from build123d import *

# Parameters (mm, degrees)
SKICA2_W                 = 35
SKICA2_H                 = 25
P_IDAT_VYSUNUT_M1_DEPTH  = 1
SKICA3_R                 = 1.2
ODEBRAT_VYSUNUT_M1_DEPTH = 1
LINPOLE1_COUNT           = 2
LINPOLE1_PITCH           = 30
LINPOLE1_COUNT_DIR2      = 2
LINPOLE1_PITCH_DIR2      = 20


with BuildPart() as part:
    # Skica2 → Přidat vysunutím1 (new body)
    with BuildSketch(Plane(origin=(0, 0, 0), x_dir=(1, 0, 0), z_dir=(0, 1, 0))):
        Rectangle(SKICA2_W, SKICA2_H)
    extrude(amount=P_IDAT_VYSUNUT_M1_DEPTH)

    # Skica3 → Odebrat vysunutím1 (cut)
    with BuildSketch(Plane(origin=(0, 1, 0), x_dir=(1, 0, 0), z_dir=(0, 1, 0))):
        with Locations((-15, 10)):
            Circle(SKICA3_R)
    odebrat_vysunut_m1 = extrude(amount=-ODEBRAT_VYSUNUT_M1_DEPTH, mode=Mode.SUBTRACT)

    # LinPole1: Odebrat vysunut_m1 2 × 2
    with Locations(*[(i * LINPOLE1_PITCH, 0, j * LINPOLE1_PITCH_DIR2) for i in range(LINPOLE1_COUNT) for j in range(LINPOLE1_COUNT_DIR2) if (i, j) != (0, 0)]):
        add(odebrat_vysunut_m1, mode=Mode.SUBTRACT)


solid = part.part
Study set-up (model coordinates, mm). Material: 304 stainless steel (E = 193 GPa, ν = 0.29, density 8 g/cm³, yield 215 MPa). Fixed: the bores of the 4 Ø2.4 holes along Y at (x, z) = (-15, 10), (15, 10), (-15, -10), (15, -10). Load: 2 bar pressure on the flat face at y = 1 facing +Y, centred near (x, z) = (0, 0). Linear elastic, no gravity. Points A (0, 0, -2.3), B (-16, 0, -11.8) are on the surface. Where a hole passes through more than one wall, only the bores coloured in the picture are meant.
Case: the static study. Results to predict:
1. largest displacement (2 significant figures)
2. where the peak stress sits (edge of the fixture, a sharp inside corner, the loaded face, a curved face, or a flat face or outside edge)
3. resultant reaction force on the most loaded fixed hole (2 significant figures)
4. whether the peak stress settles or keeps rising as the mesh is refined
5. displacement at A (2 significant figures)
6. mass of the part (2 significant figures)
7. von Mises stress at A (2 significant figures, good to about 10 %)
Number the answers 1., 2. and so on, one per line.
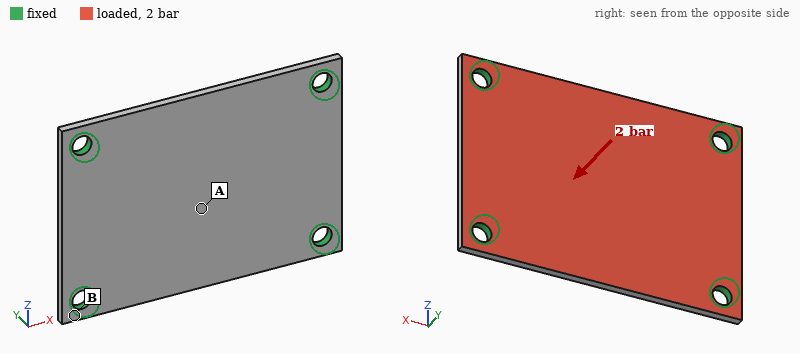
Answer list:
1. 32 µm
2. edge of the fixture
3. 43 N
4. keeps rising
5. 32 µm
6. 6.9 g
7. 41 MPa
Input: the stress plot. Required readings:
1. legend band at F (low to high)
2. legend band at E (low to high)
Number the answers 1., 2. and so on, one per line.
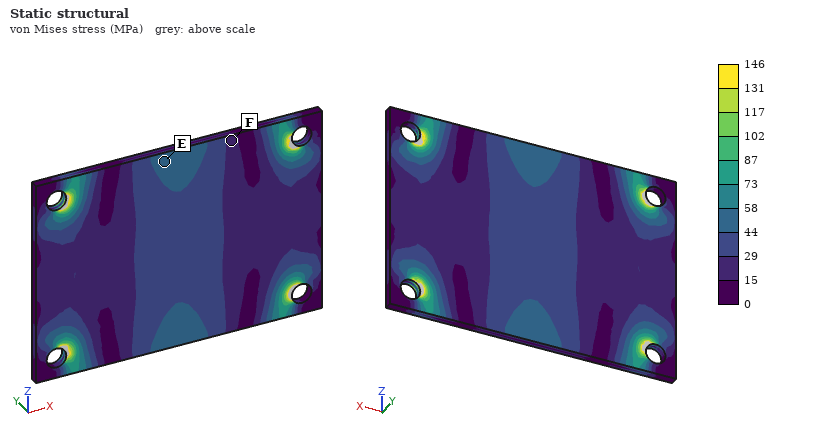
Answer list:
1. 15 to 29 MPa
2. 44 to 58 MPa
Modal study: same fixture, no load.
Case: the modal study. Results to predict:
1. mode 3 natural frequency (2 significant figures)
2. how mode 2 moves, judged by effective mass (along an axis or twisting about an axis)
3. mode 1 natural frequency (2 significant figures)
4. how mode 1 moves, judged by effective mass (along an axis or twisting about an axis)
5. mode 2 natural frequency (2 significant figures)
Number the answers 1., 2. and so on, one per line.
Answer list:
1. 12 kHz
2. twisting about X
3. 5200 Hz
4. along Y
5. 7700 Hz
